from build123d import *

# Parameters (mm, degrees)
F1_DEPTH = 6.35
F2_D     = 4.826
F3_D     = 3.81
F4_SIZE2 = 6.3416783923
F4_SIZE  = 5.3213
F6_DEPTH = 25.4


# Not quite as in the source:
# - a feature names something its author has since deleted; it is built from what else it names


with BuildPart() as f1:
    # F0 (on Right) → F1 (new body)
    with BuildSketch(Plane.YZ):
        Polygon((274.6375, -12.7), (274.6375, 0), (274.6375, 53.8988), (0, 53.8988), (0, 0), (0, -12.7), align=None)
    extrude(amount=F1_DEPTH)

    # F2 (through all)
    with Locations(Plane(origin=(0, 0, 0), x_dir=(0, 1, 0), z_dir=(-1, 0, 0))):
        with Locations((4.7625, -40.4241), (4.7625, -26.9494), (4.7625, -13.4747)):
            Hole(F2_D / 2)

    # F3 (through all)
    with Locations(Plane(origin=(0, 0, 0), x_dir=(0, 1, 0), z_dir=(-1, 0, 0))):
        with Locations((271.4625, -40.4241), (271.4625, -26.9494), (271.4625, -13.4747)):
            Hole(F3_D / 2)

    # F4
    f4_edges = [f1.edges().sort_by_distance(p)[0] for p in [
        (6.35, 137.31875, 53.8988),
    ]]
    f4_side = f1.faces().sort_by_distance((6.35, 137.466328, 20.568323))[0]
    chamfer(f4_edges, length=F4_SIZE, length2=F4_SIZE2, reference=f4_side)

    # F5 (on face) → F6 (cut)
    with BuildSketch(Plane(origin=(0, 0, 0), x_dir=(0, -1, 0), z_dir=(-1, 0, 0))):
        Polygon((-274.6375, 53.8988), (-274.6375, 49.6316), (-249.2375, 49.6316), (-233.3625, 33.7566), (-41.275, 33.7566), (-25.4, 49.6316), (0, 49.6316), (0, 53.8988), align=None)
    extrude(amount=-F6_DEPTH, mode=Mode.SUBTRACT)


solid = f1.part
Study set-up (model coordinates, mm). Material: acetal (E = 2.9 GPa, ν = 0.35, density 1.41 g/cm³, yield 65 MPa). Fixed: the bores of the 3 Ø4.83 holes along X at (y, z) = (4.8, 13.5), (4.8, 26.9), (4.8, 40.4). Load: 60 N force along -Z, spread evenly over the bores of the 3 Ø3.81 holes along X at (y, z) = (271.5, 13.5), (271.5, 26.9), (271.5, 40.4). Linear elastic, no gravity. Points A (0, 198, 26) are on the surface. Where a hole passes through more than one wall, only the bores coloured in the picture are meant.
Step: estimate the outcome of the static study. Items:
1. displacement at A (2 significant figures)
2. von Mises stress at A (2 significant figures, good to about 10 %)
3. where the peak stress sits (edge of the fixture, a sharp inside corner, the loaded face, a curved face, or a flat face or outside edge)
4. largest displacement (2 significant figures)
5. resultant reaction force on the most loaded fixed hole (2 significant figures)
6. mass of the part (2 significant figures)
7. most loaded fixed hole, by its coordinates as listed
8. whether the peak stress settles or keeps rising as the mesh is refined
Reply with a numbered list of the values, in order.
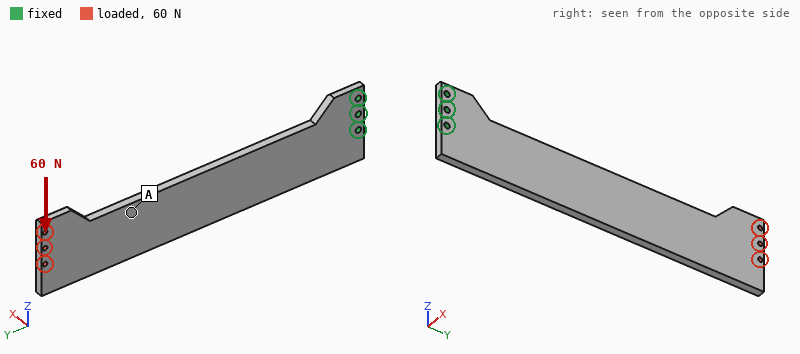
1. 1.7 mm
2. 1.3 MPa
3. edge of the fixture
4. 2.8 mm
5. 570 N
6. 120 g
7. (4.8, 13.5)
8. keeps rising
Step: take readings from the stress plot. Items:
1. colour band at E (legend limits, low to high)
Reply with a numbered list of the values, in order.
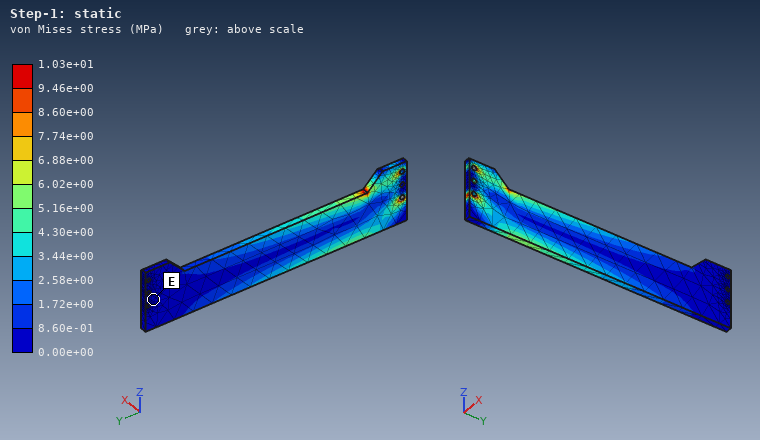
1. 0.00e+00 to 8.60e-01 MPa
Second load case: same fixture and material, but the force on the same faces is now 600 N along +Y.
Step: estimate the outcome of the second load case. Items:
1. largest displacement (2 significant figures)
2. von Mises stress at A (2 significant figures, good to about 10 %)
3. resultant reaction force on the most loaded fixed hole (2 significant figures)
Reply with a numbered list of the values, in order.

1. 2.1 mm
2. 4.9 MPa
3. 220 N
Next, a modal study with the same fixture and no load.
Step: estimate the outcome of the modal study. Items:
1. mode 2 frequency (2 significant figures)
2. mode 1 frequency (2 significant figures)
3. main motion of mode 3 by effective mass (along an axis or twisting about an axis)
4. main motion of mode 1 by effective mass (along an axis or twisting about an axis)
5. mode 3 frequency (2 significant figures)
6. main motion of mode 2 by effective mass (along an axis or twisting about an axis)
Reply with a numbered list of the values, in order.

1. 120 Hz
2. 20 Hz
3. along Z
4. along X
5. 130 Hz
6. along X
